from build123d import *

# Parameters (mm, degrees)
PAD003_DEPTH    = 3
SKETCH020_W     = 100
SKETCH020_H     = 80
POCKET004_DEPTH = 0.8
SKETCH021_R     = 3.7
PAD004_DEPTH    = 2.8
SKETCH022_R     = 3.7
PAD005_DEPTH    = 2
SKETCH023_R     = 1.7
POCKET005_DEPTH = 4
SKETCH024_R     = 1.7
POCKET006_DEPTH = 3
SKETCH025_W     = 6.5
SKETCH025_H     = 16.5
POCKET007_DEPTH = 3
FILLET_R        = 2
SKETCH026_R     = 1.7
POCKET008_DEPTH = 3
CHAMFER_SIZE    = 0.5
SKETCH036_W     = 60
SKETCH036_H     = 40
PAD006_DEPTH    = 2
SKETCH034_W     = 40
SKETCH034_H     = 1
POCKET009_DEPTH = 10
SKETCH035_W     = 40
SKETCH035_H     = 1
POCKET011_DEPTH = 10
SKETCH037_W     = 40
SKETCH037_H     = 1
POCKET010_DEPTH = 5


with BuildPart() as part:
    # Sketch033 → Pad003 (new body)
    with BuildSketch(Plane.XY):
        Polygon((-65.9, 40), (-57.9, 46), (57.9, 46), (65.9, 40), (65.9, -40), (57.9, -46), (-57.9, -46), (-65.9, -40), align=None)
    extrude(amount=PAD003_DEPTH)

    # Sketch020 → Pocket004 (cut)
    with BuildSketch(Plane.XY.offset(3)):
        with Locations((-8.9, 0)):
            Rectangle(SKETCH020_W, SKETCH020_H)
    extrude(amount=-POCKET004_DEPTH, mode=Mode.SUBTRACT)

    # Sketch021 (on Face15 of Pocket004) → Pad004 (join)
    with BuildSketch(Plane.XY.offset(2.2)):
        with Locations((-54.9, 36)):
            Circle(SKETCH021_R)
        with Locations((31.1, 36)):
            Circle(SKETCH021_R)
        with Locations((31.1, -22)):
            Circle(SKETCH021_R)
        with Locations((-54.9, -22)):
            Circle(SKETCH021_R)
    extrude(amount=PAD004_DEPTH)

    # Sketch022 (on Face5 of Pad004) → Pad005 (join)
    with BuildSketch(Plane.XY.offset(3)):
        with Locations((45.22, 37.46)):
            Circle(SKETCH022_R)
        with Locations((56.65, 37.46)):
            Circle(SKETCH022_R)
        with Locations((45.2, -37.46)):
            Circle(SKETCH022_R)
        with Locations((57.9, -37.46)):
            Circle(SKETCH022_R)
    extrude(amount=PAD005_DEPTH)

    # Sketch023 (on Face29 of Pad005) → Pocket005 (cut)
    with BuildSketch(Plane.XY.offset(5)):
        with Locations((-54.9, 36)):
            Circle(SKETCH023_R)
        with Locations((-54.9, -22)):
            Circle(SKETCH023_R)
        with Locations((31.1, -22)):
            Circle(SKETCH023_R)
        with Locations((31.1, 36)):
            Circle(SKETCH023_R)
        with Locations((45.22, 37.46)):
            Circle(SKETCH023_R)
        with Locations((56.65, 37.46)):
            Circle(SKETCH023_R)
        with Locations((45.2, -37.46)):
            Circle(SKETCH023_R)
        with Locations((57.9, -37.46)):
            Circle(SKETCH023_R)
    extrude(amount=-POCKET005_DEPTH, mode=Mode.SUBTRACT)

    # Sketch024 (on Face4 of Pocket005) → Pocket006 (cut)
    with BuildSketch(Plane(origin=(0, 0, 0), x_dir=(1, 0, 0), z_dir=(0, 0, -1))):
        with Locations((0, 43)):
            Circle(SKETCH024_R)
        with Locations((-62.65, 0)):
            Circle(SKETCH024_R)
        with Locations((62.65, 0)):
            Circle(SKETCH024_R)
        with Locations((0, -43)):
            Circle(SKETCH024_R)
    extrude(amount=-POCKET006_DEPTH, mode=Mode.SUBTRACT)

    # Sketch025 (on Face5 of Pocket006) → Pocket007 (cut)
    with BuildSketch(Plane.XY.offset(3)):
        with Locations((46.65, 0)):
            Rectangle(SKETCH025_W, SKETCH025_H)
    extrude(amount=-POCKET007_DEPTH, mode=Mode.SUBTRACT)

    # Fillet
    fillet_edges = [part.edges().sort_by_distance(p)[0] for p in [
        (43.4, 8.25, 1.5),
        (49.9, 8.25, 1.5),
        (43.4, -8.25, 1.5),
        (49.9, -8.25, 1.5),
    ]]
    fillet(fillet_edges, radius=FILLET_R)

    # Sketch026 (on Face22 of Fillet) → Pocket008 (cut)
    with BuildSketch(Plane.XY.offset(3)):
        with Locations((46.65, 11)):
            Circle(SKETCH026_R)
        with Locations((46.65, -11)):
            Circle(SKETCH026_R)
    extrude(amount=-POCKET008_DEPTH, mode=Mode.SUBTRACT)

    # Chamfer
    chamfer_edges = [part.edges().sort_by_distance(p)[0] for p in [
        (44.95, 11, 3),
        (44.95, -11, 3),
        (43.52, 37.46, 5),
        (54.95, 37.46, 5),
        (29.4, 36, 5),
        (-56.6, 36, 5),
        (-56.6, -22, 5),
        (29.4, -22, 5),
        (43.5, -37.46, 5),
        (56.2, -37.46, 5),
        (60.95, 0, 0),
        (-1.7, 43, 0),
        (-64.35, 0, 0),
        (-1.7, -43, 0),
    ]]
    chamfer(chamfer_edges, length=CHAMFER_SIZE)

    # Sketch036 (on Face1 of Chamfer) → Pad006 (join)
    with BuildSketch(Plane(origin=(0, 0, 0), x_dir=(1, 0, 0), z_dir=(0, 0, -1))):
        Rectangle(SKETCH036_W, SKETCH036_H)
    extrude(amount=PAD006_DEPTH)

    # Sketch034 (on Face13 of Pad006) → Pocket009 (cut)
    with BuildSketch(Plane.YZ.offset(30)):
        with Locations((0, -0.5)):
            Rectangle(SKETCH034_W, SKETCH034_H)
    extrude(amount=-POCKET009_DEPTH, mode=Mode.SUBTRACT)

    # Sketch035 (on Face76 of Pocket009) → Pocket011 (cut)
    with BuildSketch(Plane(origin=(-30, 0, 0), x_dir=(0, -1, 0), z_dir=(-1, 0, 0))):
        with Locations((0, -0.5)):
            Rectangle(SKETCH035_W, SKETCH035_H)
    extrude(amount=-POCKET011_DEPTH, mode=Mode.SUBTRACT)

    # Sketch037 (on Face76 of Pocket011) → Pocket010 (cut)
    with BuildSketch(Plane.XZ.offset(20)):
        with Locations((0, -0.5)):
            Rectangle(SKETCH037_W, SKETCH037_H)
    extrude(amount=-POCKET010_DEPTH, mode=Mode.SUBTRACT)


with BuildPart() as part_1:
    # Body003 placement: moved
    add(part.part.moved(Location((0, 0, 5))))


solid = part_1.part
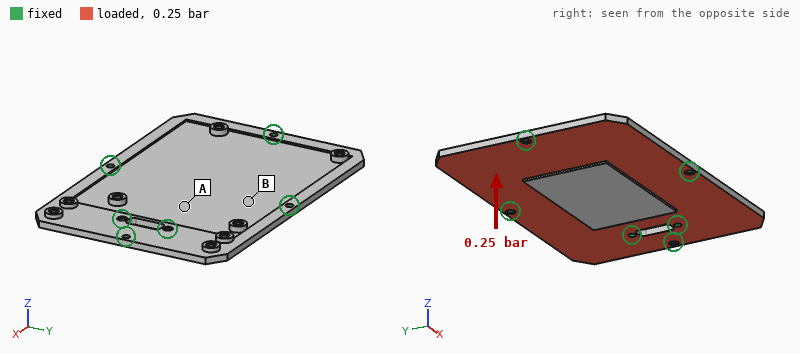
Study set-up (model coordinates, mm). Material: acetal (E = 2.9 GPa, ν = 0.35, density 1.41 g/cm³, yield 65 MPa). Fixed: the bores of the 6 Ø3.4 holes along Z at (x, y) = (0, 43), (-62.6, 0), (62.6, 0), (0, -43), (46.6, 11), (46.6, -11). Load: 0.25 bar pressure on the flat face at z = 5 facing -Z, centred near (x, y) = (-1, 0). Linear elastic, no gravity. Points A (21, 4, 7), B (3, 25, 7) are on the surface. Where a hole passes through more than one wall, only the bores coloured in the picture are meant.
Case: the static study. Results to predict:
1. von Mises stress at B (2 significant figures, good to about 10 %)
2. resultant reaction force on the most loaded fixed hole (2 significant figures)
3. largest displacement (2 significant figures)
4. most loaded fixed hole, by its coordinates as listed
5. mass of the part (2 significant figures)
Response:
4.0 MPa
80 N
1.7 mm
(-62.6, 0)
47 g
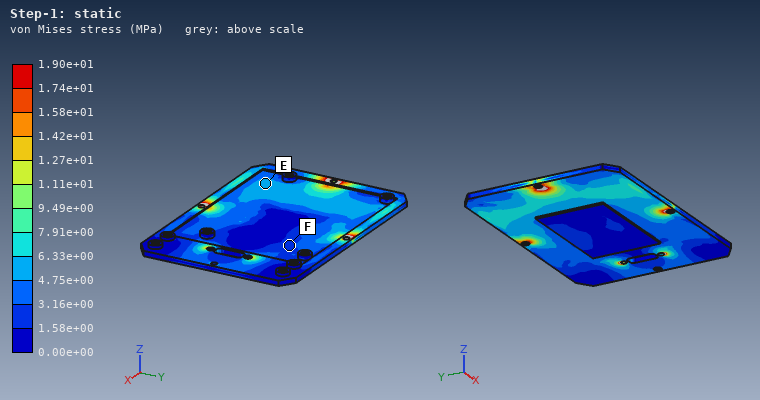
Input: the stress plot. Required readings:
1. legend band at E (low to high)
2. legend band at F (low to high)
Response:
4.75e+00 to 6.33e+00 MPa
1.58e+00 to 3.16e+00 MPa
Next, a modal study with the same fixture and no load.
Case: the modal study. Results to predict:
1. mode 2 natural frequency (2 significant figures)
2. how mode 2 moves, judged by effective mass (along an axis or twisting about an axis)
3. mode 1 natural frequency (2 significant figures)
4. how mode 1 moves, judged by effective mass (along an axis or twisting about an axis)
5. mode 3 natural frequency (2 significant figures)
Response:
410 Hz
along Z
390 Hz
twisting about X
530 Hz
